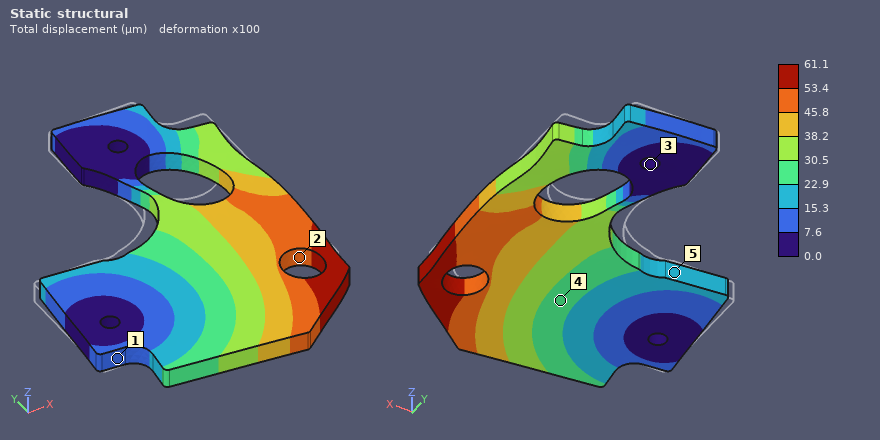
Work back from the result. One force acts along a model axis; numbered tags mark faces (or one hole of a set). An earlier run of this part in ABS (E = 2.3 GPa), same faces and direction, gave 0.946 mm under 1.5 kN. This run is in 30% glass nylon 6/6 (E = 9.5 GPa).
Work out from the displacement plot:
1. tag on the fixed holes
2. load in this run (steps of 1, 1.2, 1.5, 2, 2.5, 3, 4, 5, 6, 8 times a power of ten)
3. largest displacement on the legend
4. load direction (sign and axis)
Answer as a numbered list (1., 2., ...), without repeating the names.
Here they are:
1. 3
2. 400 N
3. 61.1 µm
4. -Y
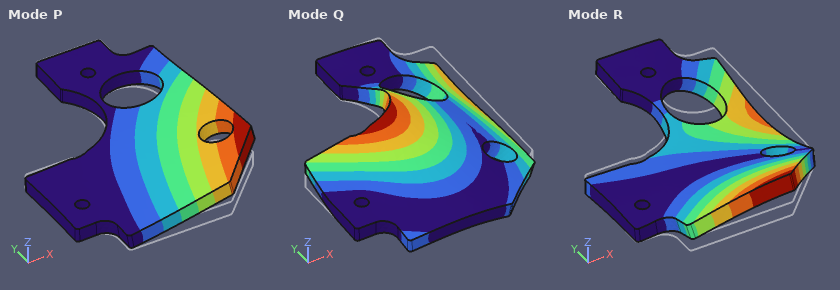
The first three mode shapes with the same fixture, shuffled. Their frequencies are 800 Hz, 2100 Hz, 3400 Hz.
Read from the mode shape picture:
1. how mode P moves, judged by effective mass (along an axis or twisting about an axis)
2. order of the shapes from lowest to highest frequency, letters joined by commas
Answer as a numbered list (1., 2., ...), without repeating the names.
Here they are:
1. along Z
2. P, R, Q
